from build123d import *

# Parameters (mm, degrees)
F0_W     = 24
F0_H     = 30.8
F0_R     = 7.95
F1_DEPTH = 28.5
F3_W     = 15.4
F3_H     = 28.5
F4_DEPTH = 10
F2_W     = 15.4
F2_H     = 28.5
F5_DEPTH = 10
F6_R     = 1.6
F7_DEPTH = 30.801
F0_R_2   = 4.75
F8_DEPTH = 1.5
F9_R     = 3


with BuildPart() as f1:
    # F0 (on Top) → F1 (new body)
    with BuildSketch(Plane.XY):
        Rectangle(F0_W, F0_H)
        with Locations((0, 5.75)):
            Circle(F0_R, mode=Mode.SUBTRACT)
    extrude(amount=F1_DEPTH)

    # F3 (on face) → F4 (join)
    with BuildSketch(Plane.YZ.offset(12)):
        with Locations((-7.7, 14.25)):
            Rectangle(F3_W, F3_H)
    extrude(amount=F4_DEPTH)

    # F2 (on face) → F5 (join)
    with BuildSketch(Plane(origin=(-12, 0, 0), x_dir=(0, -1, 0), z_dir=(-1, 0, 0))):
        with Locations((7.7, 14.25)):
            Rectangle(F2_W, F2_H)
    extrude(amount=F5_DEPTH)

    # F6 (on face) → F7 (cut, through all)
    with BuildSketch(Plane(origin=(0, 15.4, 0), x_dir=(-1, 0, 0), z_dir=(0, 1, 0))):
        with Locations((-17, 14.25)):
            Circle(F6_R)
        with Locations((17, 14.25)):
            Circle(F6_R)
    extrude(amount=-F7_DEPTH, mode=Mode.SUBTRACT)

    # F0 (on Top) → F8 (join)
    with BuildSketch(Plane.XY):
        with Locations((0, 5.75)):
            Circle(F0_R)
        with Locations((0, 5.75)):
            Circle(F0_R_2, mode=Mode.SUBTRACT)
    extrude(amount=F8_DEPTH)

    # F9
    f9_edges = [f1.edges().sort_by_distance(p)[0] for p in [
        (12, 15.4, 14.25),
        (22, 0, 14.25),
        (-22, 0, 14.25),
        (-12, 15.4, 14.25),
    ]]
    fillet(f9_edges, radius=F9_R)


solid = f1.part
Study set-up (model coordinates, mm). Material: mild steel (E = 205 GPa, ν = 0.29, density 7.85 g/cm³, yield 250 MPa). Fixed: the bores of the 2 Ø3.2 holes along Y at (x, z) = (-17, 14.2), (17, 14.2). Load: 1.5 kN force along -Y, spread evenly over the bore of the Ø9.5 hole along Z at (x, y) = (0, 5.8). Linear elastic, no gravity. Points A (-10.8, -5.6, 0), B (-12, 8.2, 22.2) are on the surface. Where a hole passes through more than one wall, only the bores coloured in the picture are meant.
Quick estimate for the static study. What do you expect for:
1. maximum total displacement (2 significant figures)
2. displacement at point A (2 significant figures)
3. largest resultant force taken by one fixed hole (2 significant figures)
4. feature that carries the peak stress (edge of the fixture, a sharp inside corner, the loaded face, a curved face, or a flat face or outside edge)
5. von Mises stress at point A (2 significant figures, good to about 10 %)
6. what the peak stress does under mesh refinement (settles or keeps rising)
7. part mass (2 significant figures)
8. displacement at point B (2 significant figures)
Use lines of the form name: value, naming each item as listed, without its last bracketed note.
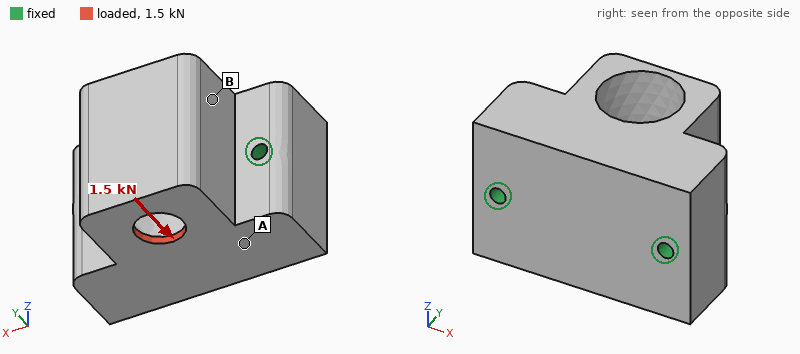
maximum total displacement: 5.5 µm
displacement at point A: 1.7 µm
largest resultant force taken by one fixed hole: 760 N
feature that carries the peak stress: a sharp inside corner
von Mises stress at point A: 11 MPa
what the peak stress does under mesh refinement: keeps rising
part mass: 190 g
displacement at point B: 1.5 µm
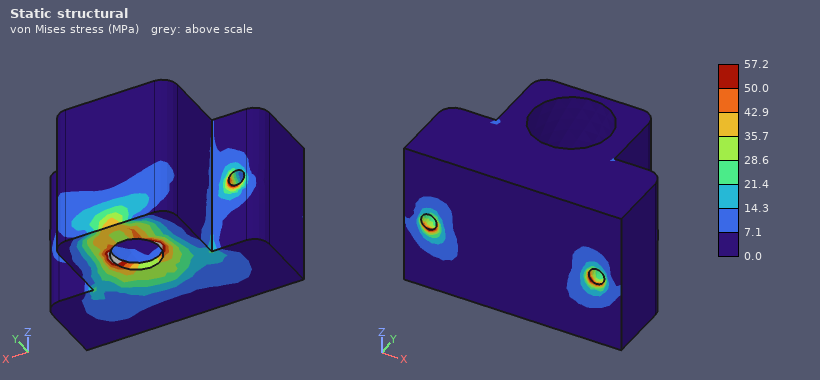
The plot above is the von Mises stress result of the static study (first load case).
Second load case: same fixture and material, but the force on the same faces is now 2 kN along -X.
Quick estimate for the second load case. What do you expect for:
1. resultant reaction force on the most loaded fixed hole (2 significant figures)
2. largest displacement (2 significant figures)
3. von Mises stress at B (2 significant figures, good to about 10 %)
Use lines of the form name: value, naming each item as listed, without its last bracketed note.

resultant reaction force on the most loaded fixed hole: 1.5 kN
largest displacement: 7.2 µm
von Mises stress at B: 7.2 MPa
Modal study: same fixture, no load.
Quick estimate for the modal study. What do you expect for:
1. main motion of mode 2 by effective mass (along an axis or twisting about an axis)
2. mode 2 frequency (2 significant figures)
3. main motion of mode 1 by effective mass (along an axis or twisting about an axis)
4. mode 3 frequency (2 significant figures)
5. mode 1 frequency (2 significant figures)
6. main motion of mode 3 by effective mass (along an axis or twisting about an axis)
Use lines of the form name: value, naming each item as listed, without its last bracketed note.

main motion of mode 2 by effective mass: along X
mode 2 frequency: 16 kHz
main motion of mode 1 by effective mass: along Z
mode 3 frequency: 23 kHz
mode 1 frequency: 14 kHz
main motion of mode 3 by effective mass: along Y
